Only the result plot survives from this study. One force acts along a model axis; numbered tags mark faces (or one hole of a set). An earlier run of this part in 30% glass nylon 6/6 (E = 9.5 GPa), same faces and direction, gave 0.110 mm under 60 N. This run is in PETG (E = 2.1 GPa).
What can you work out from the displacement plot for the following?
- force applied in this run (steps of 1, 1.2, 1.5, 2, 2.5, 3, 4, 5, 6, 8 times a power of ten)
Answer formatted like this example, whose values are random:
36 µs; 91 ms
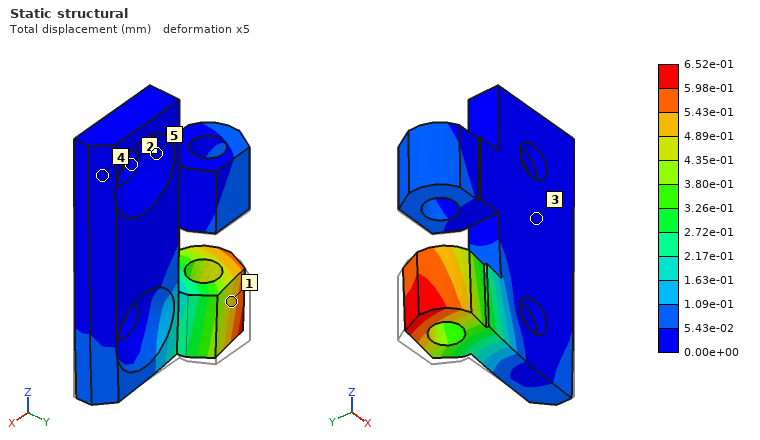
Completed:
80 N
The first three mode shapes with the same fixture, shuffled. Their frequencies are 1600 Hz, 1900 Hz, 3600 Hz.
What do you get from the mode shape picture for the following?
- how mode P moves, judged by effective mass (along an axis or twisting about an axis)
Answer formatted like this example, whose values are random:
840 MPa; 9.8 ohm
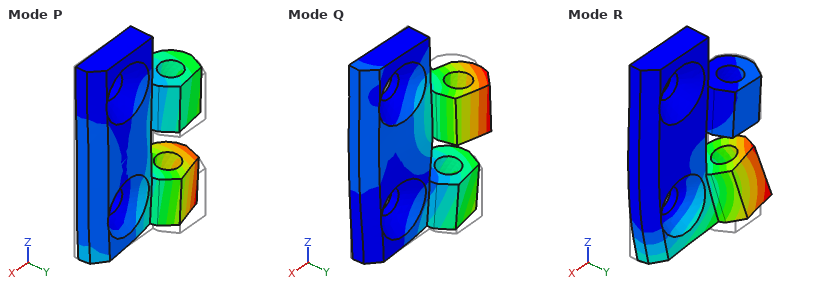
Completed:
along Y
